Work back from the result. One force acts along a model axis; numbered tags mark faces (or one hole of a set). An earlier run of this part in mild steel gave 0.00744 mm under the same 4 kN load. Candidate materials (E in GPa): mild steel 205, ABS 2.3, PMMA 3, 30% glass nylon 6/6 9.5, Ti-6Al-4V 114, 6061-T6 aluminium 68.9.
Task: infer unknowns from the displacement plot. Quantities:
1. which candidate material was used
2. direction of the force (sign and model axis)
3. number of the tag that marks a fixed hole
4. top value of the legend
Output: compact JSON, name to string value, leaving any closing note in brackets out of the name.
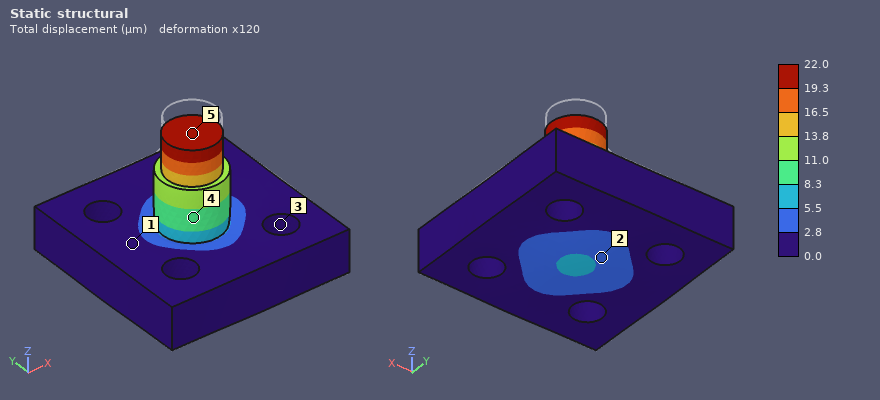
{"which candidate material was used": "6061-T6 aluminium", "direction of the force": "-Z", "number of the tag that marks a fixed hole": "3", "top value of the legend": "22.0 µm"}
